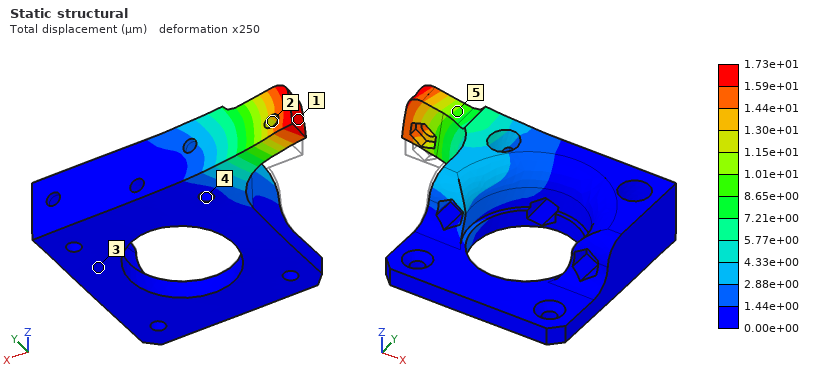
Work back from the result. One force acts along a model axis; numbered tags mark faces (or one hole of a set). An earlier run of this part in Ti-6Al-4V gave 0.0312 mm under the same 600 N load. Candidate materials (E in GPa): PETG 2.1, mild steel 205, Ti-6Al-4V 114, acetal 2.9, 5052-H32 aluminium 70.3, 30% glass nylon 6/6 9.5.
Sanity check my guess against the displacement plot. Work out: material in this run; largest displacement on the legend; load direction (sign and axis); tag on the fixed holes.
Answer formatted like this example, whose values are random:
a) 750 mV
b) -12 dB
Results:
a) mild steel
b) 1.73e+01 µm
c) +Z
d) 4
